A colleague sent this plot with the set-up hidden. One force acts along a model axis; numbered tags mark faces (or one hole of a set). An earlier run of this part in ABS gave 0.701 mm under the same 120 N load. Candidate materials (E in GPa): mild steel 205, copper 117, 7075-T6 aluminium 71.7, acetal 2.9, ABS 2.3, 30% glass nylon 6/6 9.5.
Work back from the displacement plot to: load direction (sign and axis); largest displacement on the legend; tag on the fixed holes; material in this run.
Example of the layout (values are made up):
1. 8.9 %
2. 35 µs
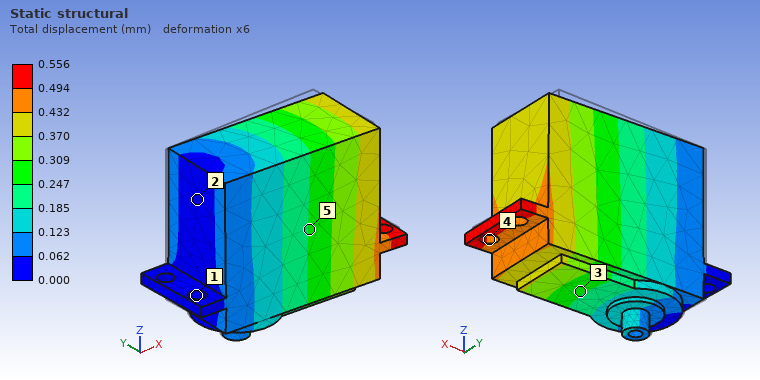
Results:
1. -Y
2. 0.556 mm
3. 1
4. acetal
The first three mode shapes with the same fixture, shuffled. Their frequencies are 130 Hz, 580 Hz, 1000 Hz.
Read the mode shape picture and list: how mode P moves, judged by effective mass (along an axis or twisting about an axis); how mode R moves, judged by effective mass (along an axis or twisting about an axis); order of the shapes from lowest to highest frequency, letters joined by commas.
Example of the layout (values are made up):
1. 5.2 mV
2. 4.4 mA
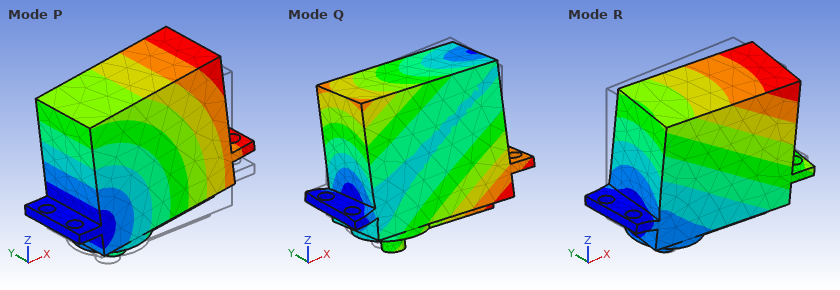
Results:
1. along Z
2. along Y
3. P, R, Q
